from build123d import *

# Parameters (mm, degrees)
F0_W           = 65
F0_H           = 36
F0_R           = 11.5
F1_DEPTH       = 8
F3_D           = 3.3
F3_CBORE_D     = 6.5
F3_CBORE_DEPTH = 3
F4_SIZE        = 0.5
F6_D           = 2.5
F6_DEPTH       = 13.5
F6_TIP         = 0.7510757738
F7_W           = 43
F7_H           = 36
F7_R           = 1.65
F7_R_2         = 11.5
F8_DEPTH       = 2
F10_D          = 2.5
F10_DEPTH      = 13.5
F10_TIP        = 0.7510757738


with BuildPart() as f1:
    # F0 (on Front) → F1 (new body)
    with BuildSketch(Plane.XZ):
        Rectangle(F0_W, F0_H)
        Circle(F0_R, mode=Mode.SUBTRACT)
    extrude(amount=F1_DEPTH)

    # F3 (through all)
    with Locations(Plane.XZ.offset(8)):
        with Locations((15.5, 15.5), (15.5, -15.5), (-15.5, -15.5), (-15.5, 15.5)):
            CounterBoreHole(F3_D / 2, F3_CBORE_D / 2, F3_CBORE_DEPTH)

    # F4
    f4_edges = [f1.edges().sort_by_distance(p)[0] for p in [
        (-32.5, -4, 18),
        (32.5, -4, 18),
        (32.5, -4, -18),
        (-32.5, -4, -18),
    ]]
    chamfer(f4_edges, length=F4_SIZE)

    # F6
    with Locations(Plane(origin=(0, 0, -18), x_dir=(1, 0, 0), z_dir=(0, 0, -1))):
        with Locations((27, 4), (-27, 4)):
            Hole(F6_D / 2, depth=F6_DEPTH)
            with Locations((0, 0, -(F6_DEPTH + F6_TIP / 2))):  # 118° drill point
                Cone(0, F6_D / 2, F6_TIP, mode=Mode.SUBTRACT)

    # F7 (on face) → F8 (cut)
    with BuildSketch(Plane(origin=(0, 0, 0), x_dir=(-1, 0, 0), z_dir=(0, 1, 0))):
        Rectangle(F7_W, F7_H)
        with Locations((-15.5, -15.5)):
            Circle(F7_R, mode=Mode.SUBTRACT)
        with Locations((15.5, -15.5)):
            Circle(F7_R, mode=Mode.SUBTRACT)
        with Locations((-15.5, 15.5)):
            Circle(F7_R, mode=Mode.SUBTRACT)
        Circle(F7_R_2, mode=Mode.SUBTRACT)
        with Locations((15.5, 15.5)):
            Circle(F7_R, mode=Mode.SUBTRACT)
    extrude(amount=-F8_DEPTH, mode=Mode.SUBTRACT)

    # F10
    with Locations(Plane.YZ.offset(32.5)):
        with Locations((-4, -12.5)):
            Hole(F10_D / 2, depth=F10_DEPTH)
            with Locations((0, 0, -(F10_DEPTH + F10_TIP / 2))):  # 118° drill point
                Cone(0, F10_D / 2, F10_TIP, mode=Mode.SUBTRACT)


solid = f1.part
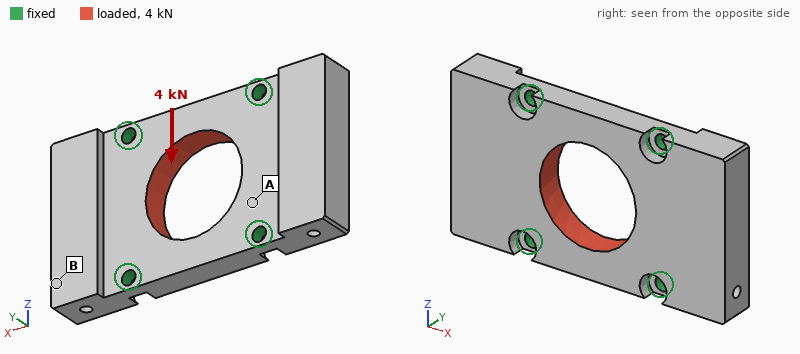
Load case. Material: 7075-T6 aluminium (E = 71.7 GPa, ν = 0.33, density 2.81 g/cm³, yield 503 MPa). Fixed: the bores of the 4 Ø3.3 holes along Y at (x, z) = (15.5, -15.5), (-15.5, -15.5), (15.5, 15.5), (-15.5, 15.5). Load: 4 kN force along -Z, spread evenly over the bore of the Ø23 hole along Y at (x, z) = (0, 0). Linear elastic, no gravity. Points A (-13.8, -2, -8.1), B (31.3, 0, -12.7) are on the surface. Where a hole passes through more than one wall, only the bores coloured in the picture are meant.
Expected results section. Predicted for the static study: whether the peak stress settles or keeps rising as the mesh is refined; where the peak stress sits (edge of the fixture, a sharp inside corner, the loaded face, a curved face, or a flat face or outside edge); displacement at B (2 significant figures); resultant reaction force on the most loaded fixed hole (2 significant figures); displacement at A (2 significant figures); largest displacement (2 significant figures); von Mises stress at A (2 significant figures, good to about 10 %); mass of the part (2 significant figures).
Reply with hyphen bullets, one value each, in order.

- keeps rising
- edge of the fixture
- 2.2 µm
- 1.0 kN
- 3.1 µm
- 11 µm
- 27 MPa
- 35 g
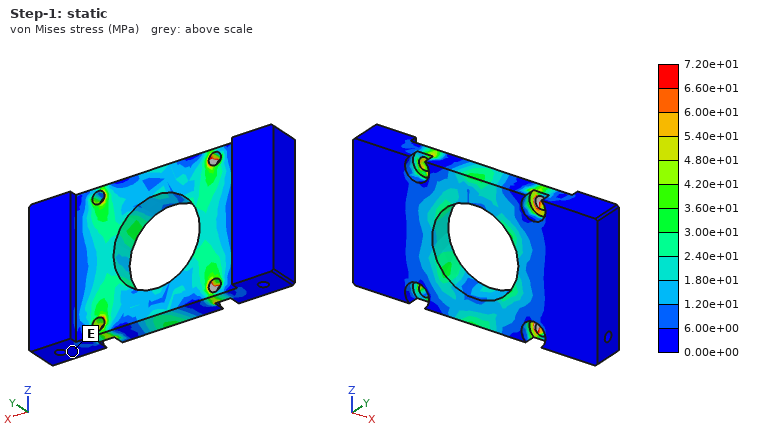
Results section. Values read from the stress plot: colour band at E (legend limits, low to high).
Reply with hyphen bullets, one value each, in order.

- 0.00e+00 to 6.00e+00 MPa
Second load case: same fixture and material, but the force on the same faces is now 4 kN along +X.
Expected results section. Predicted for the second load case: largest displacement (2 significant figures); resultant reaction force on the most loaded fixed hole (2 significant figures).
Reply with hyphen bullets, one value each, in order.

- 9.0 µm
- 1.0 kN
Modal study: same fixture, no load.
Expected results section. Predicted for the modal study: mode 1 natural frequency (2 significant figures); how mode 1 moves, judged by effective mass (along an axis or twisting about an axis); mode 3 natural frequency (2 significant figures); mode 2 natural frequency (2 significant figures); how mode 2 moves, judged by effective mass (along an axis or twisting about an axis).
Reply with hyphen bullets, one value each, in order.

- 7100 Hz
- along Y
- 18 kHz
- 7600 Hz
- twisting about Z
